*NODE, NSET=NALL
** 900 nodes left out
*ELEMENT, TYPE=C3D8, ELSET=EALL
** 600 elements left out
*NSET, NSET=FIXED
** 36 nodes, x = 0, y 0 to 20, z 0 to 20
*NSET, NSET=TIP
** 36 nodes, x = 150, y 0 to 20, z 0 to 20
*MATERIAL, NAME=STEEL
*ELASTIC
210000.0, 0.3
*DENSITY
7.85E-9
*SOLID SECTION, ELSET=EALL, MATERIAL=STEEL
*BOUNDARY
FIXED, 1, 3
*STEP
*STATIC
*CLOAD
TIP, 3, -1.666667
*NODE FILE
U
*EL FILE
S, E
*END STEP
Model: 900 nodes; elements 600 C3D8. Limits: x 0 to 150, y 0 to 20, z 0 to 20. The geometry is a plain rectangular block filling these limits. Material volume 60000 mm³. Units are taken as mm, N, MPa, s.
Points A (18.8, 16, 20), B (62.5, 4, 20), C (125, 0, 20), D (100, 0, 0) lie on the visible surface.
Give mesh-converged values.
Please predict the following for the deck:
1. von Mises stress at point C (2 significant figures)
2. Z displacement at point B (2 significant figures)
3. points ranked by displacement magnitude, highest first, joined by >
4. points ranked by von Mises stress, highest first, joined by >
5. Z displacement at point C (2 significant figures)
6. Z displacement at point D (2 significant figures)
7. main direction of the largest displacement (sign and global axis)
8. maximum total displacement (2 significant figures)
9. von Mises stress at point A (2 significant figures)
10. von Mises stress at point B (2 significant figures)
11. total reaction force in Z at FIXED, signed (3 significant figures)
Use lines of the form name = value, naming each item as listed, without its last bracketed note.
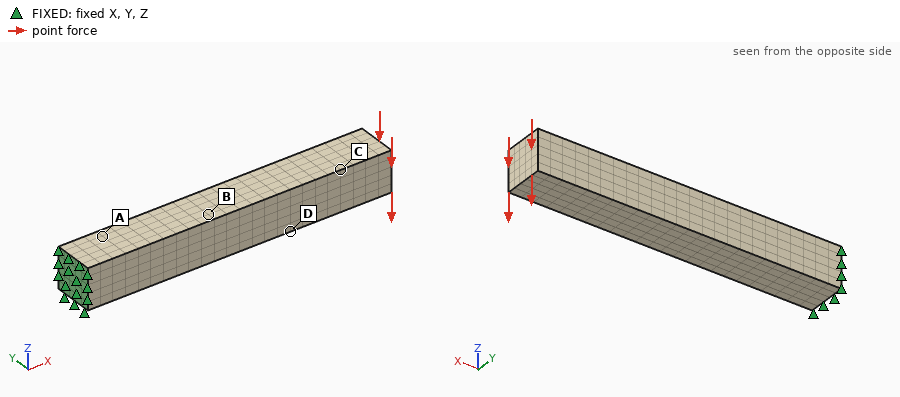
von Mises stress at point C = 1.1 MPa
Z displacement at point B = -0.0055 mm
points ranked by displacement magnitude, highest first, joined by > = C > D > B > A
points ranked by von Mises stress, highest first, joined by > = A > B > D > C
Z displacement at point C = -0.018 mm
Z displacement at point D = -0.013 mm
main direction of the largest displacement = -Z
maximum total displacement = 0.024 mm
von Mises stress at point A = 5.9 MPa
von Mises stress at point B = 3.9 MPa
total reaction force in Z at FIXED, signed = 60.0 N
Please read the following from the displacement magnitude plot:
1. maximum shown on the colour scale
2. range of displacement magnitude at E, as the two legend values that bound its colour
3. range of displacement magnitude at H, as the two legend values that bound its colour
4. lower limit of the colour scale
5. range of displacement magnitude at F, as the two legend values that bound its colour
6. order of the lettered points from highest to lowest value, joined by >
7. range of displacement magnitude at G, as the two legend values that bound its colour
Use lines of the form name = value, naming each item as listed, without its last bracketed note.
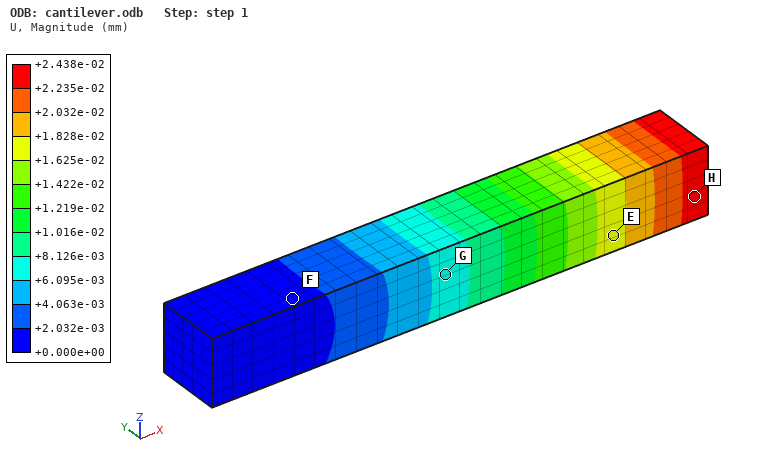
maximum shown on the colour scale = +2.438e-02 mm
range of displacement magnitude at E, as the two legend values that bound its colour = +1.625e-02 to +1.828e-02 mm
range of displacement magnitude at H, as the two legend values that bound its colour = +2.235e-02 to +2.438e-02 mm
lower limit of the colour scale = +0.000e+00 mm
range of displacement magnitude at F, as the two legend values that bound its colour = +0.000e+00 to +2.032e-03 mm
order of the lettered points from highest to lowest value, joined by > = H > E > G > F
range of displacement magnitude at G, as the two legend values that bound its colour = +6.095e-03 to +8.126e-03 mm
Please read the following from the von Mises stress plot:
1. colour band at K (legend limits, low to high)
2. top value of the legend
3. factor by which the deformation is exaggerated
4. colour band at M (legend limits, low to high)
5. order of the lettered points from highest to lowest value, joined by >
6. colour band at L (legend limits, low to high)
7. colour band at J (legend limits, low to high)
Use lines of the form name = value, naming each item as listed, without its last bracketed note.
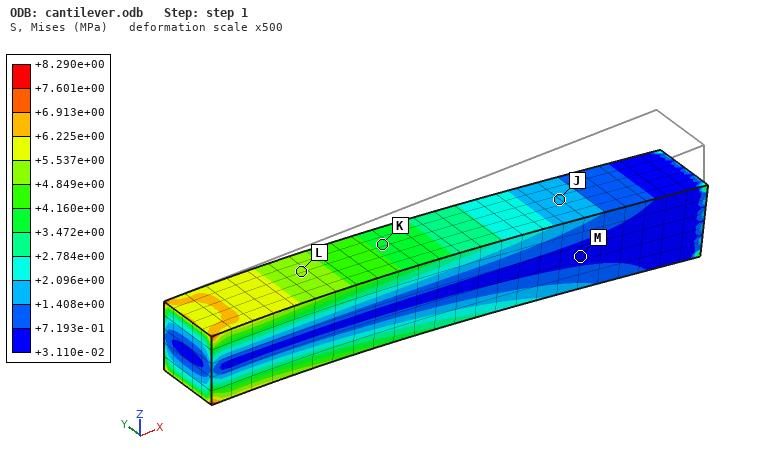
colour band at K = +3.472e+00 to +4.160e+00 MPa
top value of the legend = +8.290e+00 MPa
factor by which the deformation is exaggerated = 500
colour band at M = +3.110e-02 to +7.193e-01 MPa
order of the lettered points from highest to lowest value, joined by > = L > K > J > M
colour band at L = +4.849e+00 to +5.537e+00 MPa
colour band at J = +1.408e+00 to +2.096e+00 MPa
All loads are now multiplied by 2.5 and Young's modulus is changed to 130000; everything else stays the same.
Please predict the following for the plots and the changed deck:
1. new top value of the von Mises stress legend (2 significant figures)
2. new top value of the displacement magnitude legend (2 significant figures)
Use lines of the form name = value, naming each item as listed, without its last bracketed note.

new top value of the von Mises stress legend = 21 MPa
new top value of the displacement magnitude legend = 0.098 mm
